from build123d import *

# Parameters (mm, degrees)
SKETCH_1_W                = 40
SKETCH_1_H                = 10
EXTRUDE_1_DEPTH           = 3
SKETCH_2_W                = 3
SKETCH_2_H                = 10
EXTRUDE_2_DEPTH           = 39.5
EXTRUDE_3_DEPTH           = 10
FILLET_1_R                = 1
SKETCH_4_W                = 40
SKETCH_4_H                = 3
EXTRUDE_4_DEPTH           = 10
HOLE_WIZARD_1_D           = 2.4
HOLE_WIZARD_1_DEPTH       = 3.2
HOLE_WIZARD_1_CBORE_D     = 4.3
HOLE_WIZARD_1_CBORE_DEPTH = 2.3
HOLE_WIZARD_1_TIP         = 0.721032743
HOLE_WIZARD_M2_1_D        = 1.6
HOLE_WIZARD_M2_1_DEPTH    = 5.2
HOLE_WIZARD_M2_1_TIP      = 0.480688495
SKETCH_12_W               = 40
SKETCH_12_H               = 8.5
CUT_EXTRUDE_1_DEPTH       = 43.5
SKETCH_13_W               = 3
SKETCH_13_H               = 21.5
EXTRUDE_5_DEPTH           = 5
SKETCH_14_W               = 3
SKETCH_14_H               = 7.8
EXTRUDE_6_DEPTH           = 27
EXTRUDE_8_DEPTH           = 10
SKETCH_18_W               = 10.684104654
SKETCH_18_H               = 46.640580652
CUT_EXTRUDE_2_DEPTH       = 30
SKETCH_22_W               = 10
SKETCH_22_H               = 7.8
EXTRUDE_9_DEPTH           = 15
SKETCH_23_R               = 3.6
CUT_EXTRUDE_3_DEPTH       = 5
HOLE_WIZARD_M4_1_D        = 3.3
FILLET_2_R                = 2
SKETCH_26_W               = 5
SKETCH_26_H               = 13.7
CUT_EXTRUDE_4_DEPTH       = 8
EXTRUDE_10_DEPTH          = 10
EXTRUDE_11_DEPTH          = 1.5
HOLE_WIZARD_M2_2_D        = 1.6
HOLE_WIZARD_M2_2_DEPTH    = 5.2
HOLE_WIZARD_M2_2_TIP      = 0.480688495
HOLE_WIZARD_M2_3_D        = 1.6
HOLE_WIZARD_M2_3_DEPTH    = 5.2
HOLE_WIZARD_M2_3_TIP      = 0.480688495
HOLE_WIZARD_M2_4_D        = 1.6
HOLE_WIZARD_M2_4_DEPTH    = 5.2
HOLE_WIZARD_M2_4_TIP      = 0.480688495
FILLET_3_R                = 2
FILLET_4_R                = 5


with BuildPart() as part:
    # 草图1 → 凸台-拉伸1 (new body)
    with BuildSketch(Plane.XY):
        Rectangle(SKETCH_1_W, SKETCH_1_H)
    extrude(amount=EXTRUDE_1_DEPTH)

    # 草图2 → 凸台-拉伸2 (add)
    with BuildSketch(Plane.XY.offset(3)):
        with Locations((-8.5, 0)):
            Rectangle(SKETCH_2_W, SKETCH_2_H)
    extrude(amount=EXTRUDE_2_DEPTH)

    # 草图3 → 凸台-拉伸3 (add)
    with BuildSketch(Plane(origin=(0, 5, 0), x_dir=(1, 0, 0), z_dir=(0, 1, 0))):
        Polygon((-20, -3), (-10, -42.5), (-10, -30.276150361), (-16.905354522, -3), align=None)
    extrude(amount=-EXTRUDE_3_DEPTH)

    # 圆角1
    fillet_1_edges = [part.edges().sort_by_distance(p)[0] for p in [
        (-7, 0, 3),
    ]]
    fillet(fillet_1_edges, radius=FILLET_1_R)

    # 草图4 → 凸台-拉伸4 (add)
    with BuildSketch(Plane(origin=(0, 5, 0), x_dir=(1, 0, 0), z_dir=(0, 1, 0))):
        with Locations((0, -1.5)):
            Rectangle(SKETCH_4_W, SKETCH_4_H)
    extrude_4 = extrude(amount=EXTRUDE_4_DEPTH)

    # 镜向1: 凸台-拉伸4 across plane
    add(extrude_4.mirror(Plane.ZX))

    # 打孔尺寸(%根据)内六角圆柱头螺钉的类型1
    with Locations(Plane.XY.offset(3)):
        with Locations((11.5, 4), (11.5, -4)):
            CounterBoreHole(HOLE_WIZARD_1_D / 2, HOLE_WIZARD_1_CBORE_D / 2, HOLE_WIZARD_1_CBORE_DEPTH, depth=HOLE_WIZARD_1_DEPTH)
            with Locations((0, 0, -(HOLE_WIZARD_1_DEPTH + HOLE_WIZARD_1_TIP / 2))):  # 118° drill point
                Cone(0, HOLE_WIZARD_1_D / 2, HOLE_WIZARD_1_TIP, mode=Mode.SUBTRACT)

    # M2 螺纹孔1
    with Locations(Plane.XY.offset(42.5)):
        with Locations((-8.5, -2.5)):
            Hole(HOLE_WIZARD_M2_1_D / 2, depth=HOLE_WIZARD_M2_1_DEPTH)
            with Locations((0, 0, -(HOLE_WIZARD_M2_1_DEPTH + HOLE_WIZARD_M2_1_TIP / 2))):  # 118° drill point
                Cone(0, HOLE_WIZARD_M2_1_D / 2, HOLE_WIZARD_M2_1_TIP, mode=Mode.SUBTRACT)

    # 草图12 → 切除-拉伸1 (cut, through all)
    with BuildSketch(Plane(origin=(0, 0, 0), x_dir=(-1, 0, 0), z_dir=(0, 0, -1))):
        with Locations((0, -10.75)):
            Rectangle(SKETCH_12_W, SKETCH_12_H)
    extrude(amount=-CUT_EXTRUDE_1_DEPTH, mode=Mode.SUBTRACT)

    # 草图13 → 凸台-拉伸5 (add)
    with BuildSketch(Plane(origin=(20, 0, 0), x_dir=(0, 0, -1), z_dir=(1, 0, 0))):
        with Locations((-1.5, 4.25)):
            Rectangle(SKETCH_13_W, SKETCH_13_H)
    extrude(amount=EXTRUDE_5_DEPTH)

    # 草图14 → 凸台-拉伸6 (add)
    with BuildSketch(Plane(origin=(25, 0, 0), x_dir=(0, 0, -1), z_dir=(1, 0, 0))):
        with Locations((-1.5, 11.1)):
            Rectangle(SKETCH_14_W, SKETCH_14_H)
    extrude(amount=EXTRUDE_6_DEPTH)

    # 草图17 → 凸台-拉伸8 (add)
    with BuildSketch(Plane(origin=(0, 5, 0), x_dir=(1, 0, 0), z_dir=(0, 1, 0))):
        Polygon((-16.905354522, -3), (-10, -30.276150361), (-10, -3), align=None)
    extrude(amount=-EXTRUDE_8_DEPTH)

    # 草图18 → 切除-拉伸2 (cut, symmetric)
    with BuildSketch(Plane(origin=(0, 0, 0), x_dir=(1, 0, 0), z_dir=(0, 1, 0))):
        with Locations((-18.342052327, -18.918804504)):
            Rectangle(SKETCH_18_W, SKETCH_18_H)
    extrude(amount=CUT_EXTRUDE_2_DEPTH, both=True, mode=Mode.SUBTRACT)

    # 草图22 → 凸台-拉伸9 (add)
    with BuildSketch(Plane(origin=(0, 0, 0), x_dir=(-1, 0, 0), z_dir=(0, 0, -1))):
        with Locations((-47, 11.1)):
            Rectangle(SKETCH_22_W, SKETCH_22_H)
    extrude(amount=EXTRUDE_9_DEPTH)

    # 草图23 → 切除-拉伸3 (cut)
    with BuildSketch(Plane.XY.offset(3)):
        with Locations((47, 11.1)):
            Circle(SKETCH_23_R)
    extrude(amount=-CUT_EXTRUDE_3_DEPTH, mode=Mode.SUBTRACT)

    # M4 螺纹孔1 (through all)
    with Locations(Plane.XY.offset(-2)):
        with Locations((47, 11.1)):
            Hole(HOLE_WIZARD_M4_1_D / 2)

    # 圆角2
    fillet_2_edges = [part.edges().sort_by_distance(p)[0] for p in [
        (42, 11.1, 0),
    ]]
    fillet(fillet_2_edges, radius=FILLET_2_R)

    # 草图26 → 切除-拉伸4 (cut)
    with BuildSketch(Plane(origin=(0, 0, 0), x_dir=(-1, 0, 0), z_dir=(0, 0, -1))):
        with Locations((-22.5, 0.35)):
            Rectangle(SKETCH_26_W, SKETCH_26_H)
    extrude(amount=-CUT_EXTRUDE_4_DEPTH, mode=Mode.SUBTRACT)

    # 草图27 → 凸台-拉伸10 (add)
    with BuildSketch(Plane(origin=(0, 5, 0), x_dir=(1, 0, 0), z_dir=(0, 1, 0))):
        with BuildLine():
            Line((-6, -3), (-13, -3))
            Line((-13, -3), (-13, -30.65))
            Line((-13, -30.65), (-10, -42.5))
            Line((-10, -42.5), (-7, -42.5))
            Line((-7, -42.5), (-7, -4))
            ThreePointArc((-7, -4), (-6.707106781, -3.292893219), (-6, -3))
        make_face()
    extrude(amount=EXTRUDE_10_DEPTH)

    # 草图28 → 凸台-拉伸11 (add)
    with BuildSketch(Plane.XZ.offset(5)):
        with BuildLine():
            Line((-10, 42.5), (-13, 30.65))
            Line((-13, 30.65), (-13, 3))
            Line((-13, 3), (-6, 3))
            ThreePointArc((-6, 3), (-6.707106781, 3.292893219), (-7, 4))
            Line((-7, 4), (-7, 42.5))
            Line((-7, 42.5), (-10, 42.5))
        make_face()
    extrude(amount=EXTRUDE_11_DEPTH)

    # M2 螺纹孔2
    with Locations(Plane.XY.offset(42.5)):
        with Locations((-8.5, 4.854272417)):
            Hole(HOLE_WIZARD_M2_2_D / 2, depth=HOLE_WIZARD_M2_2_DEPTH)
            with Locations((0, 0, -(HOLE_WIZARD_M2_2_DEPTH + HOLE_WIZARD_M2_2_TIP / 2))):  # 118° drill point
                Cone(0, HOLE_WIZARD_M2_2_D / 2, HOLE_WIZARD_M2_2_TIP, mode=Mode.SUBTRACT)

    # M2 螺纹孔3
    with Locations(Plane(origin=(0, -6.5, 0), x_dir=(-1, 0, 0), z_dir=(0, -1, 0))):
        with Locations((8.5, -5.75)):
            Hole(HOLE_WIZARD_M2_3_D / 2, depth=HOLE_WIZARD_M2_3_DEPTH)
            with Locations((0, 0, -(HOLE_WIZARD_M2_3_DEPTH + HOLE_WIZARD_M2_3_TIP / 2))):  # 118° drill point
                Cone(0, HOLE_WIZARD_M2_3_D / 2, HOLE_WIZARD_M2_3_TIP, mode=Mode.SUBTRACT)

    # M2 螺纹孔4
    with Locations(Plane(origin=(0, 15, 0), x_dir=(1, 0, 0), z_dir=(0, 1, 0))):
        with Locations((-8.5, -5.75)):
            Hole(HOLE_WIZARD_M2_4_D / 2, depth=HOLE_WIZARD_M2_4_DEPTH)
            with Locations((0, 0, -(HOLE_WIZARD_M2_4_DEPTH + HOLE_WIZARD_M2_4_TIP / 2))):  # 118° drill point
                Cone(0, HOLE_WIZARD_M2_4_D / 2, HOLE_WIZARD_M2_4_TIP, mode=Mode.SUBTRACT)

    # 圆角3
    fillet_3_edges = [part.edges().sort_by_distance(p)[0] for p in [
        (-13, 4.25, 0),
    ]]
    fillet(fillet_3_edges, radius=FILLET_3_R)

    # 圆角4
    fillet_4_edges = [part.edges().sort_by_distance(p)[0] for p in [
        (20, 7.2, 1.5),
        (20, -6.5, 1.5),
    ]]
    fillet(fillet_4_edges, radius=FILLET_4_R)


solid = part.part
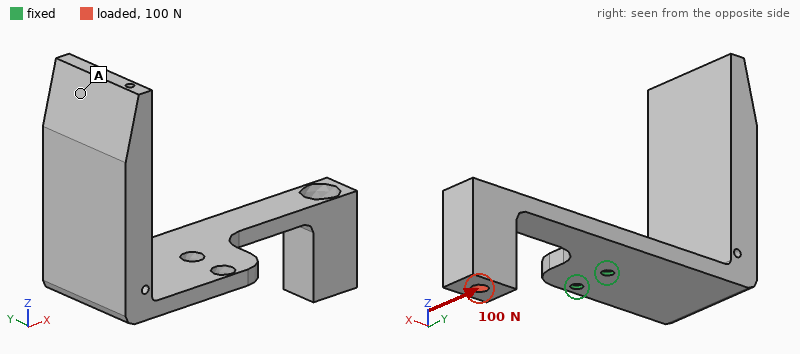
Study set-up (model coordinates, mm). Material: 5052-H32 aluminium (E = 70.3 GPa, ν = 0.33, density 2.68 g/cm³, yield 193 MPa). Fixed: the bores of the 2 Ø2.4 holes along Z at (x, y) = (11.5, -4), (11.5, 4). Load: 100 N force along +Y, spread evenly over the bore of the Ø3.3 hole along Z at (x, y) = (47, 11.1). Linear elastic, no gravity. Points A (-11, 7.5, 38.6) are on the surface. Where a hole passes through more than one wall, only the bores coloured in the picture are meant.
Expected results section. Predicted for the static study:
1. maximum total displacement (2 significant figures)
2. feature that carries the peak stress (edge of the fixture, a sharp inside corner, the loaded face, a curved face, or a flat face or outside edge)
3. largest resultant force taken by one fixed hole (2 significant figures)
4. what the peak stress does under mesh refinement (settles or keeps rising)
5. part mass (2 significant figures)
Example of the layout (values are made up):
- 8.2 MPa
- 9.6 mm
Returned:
- 0.50 mm
- edge of the fixture
- 400 N
- keeps rising
- 22 g
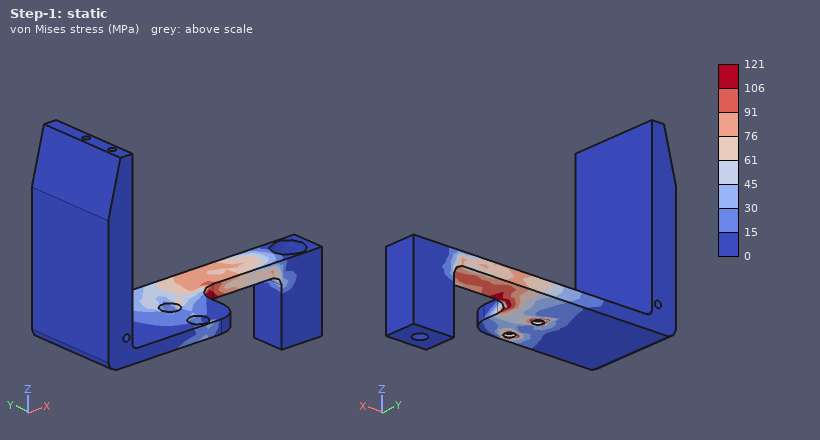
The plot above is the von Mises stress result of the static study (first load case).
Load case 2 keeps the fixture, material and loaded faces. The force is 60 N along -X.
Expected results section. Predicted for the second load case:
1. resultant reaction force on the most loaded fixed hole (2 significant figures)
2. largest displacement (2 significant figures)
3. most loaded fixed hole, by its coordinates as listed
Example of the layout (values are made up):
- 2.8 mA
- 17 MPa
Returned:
- 110 N
- 0.51 mm
- (11.5, 4)
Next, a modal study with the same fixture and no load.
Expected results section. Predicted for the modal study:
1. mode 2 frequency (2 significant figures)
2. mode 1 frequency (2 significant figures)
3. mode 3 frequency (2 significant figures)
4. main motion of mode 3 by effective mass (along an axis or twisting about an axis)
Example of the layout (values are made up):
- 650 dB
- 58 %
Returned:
- 800 Hz
- 430 Hz
- 990 Hz
- along Y
